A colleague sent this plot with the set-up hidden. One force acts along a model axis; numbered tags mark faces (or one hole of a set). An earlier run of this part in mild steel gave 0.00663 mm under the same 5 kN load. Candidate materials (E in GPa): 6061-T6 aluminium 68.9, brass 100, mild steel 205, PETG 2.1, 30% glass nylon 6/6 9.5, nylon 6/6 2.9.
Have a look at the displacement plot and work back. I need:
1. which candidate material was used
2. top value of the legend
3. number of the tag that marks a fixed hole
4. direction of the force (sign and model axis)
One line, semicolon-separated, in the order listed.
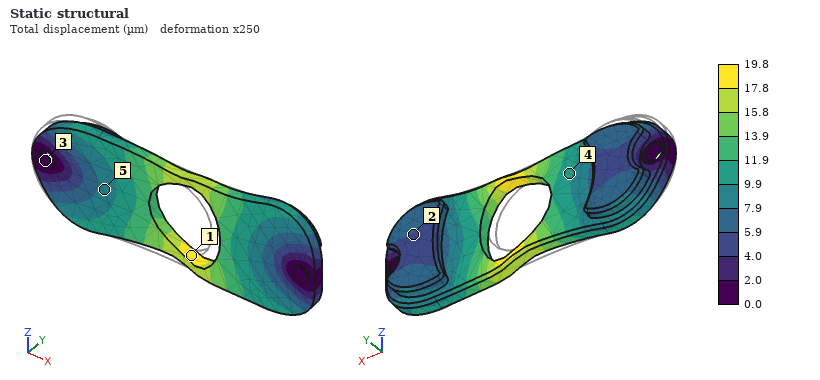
6061-T6 aluminium; 19.8 µm; 3; +X
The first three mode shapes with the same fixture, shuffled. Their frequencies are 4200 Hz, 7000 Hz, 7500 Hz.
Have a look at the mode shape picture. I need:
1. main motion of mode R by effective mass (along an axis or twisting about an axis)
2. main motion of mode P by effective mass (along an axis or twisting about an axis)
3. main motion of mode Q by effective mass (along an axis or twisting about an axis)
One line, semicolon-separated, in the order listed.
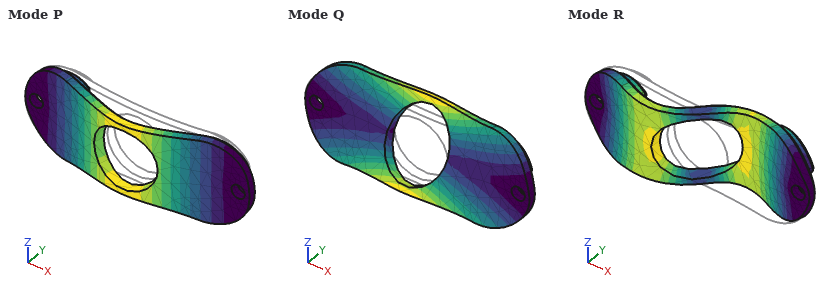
twisting about Z; along Y; twisting about X
